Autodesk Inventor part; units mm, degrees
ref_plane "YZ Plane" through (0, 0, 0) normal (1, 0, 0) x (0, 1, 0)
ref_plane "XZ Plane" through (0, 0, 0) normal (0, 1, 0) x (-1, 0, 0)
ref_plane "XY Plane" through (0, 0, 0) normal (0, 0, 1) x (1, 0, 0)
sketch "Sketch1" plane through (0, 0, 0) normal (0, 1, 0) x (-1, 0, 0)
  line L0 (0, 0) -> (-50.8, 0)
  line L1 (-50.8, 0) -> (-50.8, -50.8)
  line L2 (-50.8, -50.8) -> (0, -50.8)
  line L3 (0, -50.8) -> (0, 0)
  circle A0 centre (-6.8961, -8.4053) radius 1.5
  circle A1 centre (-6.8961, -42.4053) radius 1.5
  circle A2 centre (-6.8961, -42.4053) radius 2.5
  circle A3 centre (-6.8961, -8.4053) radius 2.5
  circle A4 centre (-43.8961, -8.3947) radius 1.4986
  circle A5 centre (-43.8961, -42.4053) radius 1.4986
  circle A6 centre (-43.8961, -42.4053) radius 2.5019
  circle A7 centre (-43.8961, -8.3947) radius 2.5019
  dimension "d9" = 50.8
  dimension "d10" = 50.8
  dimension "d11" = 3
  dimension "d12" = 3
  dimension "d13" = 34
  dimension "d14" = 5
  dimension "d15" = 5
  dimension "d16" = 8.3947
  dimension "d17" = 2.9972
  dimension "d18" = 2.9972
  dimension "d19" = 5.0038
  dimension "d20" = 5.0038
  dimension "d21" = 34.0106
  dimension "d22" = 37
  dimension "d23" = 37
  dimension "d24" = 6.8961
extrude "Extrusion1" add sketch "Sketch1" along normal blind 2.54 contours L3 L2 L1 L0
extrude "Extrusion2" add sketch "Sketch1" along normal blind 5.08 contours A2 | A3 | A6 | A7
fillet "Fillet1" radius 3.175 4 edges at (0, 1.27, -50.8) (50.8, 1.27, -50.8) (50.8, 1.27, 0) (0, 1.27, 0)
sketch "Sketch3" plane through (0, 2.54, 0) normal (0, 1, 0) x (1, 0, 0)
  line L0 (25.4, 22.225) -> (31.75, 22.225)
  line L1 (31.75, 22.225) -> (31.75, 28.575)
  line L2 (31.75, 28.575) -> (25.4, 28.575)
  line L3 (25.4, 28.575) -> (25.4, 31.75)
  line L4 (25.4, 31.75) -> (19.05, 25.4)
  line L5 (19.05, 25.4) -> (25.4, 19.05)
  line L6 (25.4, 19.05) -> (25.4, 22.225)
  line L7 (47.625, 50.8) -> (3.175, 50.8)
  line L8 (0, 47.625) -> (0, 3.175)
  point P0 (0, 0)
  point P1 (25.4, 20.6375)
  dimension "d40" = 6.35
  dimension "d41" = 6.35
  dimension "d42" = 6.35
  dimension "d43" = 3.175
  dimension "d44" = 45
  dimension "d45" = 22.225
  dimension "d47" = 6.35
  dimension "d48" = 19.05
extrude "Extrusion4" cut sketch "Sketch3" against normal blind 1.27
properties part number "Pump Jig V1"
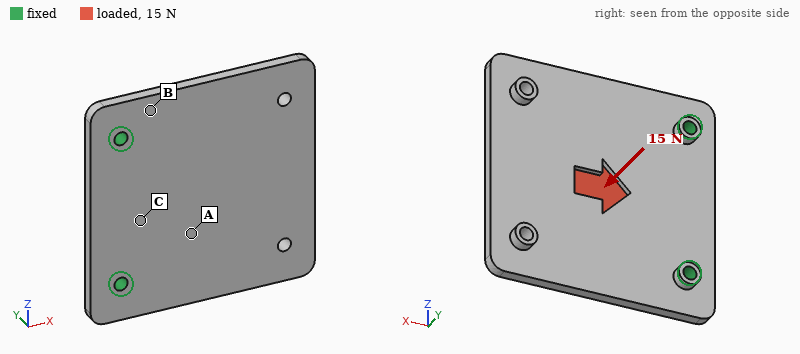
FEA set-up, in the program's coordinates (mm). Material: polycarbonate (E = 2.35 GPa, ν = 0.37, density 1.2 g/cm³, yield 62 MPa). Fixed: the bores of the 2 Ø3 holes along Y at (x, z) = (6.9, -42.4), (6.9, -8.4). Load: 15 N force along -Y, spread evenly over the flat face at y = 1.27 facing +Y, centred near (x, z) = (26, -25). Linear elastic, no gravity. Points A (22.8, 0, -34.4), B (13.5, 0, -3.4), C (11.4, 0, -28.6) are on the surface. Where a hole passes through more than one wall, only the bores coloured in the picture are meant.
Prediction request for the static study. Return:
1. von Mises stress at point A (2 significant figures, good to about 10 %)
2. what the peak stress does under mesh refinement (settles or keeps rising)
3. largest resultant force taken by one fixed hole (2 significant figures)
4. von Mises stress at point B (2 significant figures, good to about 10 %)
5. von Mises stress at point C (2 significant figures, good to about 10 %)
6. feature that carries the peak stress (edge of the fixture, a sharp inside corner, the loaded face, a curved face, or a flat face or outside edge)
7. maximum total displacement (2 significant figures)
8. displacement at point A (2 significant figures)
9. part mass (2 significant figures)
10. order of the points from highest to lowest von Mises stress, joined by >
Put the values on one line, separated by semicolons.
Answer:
0.93 MPa; keeps rising; 7.7 N; 4.1 MPa; 2.6 MPa; edge of the fixture; 0.79 mm; 0.23 mm; 7.8 g; B > C > A
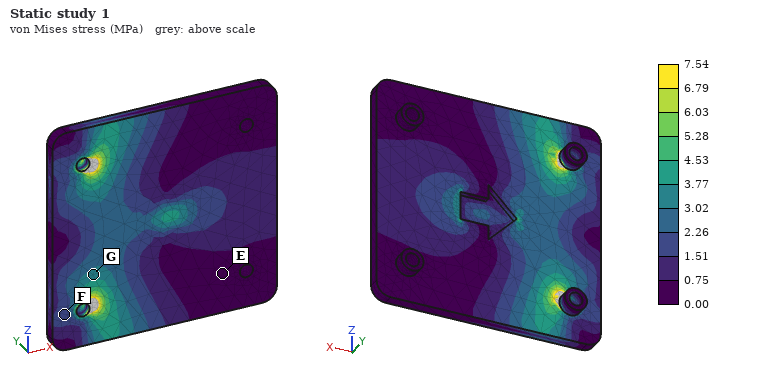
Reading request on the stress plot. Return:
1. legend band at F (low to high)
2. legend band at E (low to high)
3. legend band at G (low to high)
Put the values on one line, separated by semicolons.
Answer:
1.51 to 2.26 MPa; 0.00 to 0.75 MPa; 3.02 to 3.77 MPa
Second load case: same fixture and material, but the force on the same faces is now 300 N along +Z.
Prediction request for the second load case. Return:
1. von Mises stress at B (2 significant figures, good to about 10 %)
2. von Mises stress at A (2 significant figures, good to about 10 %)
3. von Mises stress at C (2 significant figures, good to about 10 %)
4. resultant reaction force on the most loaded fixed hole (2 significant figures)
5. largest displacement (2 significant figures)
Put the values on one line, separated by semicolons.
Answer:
2.6 MPa; 6.3 MPa; 3.8 MPa; 220 N; 0.14 mm
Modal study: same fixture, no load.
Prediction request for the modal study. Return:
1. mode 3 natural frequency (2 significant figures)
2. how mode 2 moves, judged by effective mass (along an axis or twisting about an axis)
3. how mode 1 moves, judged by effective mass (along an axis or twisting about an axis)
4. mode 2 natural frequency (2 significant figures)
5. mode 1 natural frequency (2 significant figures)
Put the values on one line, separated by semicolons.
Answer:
1700 Hz; twisting about X; along Y; 640 Hz; 280 Hz
